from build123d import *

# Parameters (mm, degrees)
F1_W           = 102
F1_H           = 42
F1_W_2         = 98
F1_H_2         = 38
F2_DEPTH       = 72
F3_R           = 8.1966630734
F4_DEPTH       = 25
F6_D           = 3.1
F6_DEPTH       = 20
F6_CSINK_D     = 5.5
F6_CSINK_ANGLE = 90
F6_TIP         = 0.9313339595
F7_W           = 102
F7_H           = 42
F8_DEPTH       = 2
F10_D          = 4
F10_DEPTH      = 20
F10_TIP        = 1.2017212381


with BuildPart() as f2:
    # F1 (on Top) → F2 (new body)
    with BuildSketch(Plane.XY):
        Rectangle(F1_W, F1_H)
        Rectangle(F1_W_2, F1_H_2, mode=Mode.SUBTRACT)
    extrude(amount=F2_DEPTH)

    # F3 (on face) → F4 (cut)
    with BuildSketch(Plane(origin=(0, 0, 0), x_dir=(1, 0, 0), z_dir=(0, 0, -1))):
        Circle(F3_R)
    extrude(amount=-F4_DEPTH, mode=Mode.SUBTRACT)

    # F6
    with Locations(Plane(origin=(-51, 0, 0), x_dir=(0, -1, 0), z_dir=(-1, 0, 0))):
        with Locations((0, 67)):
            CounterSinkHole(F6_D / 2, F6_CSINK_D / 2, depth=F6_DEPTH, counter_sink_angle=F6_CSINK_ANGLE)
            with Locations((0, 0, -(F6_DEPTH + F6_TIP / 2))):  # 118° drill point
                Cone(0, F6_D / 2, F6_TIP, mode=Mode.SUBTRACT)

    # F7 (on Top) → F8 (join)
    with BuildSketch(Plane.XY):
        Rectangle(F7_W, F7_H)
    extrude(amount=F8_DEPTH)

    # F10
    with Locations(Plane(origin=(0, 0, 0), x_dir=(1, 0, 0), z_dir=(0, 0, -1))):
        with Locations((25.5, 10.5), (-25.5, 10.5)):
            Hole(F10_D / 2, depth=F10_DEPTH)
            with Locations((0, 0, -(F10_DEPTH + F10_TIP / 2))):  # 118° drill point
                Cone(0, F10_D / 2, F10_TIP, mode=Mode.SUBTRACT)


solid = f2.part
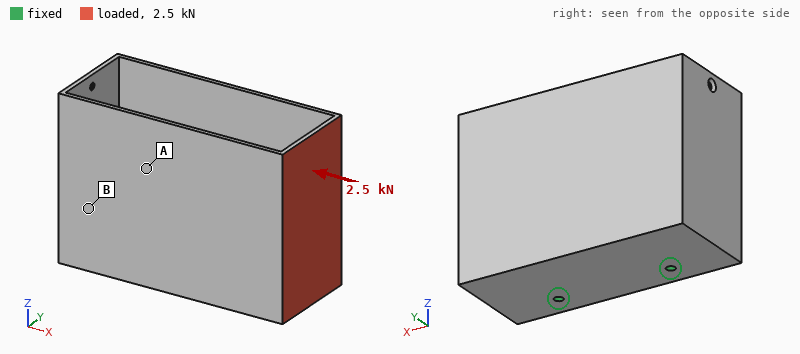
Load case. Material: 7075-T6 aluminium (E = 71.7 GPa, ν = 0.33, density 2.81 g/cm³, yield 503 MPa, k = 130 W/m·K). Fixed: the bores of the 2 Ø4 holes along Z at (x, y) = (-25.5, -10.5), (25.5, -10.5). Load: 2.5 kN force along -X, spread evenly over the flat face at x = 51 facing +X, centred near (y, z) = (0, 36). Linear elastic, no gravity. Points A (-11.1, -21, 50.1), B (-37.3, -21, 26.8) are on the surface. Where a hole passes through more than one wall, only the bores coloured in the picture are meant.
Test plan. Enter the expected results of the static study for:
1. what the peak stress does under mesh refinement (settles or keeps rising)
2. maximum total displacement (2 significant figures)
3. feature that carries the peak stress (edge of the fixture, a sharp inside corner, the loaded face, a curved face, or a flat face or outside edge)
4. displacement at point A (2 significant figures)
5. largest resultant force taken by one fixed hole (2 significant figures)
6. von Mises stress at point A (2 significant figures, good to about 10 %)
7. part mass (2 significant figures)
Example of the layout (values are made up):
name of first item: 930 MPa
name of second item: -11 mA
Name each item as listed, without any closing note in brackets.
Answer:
what the peak stress does under mesh refinement: keeps rising
maximum total displacement: 1.3 mm
feature that carries the peak stress: edge of the fixture
displacement at point A: 0.30 mm
largest resultant force taken by one fixed hole: 2.2 kN
von Mises stress at point A: 47 MPa
part mass: 130 g
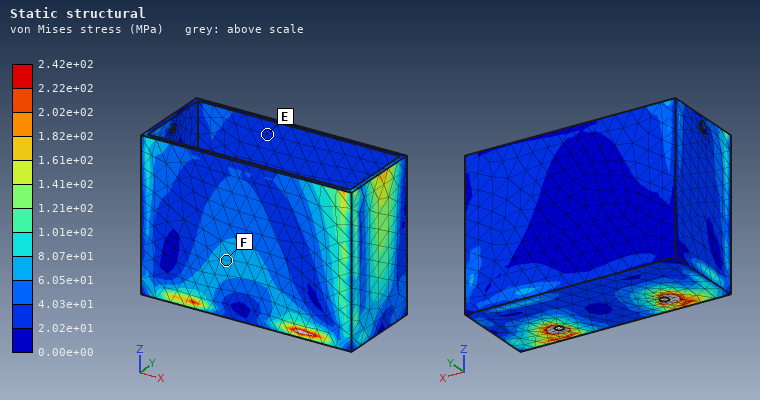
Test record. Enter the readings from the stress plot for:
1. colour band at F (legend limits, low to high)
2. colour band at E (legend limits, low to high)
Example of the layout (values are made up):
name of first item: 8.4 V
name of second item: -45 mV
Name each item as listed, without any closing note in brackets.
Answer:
colour band at F: 6.05e+01 to 8.07e+01 MPa
colour band at E: 2.02e+01 to 4.03e+01 MPa
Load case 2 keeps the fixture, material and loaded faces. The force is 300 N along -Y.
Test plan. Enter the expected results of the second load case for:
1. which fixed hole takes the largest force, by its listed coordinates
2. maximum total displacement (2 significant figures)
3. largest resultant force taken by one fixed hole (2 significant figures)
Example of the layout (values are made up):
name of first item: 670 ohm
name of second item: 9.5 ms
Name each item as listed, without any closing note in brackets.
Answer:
which fixed hole takes the largest force, by its listed coordinates: (25.5, -10.5)
maximum total displacement: 1.5 mm
largest resultant force taken by one fixed hole: 440 N
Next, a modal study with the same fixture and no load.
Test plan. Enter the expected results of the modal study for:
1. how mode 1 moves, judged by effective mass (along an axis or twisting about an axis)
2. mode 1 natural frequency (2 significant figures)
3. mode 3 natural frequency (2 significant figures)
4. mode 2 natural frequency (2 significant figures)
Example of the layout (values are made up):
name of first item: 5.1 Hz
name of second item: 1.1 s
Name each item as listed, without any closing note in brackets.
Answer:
how mode 1 moves, judged by effective mass: along Y
mode 1 natural frequency: 260 Hz
mode 3 natural frequency: 930 Hz
mode 2 natural frequency: 600 Hz
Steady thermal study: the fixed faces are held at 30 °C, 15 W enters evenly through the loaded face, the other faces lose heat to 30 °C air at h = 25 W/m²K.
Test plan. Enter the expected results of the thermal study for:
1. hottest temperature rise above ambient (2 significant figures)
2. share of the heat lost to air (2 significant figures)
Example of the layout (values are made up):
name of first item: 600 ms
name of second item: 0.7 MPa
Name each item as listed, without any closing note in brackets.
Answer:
hottest temperature rise above ambient: 20 K
share of the heat lost to air: 53 %
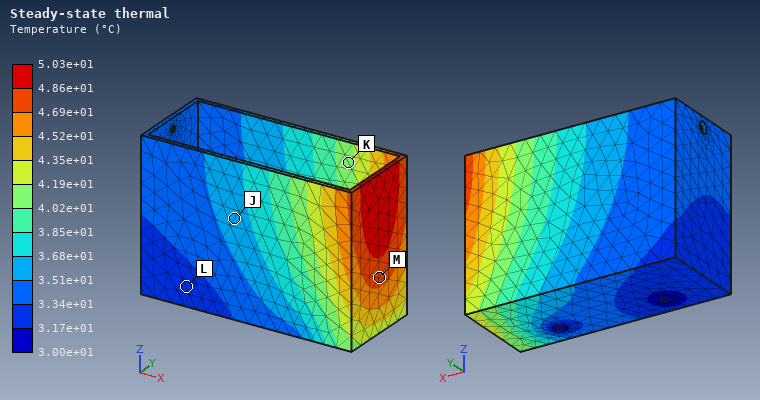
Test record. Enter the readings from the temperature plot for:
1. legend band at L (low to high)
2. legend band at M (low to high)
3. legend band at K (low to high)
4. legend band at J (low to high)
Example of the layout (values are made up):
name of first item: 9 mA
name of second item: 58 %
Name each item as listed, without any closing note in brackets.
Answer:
legend band at L: 3.17e+01 to 3.34e+01 °C
legend band at M: 4.69e+01 to 4.86e+01 °C
legend band at K: 4.02e+01 to 4.19e+01 °C
legend band at J: 3.51e+01 to 3.68e+01 °C
